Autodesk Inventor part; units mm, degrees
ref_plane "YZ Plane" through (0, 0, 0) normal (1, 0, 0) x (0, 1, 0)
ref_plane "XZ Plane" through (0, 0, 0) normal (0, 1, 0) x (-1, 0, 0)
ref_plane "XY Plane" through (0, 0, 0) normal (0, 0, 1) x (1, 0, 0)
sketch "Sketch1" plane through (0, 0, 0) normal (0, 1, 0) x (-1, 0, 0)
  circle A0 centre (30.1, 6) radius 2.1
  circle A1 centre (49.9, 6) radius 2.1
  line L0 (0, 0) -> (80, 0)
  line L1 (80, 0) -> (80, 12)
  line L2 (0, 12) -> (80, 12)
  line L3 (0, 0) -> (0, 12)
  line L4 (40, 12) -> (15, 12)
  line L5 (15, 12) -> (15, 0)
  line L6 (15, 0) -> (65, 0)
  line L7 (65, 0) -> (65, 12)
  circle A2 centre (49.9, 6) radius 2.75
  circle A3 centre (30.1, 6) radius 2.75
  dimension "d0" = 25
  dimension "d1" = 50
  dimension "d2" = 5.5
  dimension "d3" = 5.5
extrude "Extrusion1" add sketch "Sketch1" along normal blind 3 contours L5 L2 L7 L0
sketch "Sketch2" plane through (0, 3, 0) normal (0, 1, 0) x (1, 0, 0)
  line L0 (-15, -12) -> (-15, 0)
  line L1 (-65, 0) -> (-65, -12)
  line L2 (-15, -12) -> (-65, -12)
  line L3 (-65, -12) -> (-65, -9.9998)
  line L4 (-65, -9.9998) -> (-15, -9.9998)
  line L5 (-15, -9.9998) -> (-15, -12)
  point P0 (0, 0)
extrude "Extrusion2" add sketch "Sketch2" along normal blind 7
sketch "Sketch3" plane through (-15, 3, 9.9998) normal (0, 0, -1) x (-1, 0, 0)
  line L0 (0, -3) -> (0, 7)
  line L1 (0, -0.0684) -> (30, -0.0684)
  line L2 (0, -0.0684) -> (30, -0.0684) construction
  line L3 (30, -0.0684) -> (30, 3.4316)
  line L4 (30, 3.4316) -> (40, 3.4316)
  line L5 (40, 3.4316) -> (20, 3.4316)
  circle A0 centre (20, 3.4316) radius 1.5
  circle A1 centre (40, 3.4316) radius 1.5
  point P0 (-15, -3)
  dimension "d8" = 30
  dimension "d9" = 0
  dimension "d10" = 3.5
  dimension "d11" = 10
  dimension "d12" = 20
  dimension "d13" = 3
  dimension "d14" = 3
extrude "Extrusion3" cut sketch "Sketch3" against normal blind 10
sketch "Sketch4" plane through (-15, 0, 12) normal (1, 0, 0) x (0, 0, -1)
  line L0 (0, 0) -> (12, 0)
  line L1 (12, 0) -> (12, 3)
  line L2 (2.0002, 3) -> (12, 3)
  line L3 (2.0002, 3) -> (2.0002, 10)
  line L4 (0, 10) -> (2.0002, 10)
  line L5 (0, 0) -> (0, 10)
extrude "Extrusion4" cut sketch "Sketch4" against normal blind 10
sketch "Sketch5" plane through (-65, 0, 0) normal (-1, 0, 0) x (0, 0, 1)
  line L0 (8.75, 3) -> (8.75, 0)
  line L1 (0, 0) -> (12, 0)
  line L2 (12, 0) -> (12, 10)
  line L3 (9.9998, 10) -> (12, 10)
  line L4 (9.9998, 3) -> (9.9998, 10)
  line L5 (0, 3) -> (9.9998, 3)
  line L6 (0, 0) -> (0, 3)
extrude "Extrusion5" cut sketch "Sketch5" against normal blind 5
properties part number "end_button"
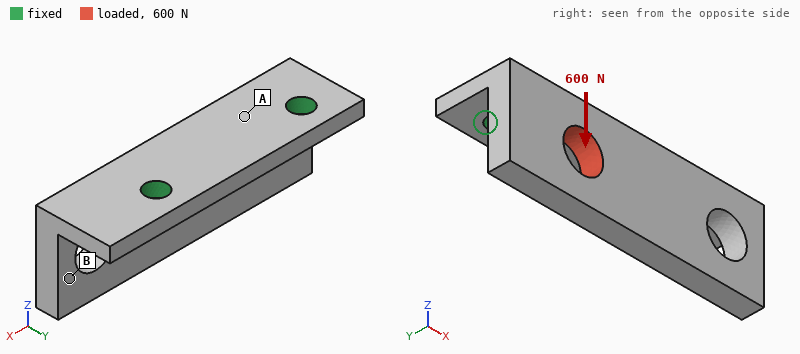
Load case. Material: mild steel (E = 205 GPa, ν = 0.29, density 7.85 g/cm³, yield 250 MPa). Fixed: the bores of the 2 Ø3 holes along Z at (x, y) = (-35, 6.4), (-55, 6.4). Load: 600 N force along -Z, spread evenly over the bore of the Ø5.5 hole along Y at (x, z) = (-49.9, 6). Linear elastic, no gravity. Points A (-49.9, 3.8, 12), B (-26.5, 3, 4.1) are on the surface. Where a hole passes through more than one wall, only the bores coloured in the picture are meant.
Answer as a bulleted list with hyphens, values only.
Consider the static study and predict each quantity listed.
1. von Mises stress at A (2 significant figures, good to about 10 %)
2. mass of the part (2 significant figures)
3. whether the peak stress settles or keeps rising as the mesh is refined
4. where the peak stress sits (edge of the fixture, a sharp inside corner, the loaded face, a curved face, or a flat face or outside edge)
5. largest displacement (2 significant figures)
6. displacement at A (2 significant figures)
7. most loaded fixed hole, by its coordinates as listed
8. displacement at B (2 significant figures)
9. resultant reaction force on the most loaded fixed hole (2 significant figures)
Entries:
- 44 MPa
- 12 g
- keeps rising
- edge of the fixture
- 25 µm
- 4.2 µm
- (-55, 6.4)
- 7.5 µm
- 440 N
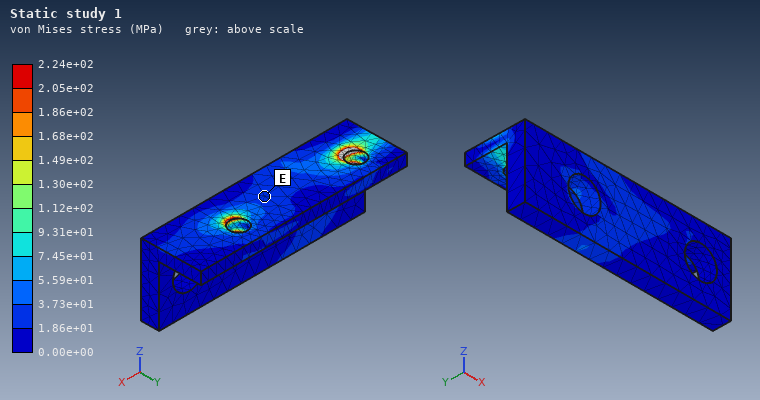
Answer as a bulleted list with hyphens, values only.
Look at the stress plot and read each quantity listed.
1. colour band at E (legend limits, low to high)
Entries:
- 1.86e+01 to 3.73e+01 MPa
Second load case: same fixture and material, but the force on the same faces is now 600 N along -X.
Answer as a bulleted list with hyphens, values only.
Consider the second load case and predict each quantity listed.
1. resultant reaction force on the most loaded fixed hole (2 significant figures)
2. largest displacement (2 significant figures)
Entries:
- 370 N
- 5.9 µm
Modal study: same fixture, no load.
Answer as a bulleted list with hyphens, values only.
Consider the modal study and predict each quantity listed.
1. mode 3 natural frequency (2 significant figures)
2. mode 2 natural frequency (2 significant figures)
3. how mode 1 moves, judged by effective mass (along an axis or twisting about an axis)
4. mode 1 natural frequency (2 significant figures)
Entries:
- 20 kHz
- 12 kHz
- along Y
- 7400 Hz
